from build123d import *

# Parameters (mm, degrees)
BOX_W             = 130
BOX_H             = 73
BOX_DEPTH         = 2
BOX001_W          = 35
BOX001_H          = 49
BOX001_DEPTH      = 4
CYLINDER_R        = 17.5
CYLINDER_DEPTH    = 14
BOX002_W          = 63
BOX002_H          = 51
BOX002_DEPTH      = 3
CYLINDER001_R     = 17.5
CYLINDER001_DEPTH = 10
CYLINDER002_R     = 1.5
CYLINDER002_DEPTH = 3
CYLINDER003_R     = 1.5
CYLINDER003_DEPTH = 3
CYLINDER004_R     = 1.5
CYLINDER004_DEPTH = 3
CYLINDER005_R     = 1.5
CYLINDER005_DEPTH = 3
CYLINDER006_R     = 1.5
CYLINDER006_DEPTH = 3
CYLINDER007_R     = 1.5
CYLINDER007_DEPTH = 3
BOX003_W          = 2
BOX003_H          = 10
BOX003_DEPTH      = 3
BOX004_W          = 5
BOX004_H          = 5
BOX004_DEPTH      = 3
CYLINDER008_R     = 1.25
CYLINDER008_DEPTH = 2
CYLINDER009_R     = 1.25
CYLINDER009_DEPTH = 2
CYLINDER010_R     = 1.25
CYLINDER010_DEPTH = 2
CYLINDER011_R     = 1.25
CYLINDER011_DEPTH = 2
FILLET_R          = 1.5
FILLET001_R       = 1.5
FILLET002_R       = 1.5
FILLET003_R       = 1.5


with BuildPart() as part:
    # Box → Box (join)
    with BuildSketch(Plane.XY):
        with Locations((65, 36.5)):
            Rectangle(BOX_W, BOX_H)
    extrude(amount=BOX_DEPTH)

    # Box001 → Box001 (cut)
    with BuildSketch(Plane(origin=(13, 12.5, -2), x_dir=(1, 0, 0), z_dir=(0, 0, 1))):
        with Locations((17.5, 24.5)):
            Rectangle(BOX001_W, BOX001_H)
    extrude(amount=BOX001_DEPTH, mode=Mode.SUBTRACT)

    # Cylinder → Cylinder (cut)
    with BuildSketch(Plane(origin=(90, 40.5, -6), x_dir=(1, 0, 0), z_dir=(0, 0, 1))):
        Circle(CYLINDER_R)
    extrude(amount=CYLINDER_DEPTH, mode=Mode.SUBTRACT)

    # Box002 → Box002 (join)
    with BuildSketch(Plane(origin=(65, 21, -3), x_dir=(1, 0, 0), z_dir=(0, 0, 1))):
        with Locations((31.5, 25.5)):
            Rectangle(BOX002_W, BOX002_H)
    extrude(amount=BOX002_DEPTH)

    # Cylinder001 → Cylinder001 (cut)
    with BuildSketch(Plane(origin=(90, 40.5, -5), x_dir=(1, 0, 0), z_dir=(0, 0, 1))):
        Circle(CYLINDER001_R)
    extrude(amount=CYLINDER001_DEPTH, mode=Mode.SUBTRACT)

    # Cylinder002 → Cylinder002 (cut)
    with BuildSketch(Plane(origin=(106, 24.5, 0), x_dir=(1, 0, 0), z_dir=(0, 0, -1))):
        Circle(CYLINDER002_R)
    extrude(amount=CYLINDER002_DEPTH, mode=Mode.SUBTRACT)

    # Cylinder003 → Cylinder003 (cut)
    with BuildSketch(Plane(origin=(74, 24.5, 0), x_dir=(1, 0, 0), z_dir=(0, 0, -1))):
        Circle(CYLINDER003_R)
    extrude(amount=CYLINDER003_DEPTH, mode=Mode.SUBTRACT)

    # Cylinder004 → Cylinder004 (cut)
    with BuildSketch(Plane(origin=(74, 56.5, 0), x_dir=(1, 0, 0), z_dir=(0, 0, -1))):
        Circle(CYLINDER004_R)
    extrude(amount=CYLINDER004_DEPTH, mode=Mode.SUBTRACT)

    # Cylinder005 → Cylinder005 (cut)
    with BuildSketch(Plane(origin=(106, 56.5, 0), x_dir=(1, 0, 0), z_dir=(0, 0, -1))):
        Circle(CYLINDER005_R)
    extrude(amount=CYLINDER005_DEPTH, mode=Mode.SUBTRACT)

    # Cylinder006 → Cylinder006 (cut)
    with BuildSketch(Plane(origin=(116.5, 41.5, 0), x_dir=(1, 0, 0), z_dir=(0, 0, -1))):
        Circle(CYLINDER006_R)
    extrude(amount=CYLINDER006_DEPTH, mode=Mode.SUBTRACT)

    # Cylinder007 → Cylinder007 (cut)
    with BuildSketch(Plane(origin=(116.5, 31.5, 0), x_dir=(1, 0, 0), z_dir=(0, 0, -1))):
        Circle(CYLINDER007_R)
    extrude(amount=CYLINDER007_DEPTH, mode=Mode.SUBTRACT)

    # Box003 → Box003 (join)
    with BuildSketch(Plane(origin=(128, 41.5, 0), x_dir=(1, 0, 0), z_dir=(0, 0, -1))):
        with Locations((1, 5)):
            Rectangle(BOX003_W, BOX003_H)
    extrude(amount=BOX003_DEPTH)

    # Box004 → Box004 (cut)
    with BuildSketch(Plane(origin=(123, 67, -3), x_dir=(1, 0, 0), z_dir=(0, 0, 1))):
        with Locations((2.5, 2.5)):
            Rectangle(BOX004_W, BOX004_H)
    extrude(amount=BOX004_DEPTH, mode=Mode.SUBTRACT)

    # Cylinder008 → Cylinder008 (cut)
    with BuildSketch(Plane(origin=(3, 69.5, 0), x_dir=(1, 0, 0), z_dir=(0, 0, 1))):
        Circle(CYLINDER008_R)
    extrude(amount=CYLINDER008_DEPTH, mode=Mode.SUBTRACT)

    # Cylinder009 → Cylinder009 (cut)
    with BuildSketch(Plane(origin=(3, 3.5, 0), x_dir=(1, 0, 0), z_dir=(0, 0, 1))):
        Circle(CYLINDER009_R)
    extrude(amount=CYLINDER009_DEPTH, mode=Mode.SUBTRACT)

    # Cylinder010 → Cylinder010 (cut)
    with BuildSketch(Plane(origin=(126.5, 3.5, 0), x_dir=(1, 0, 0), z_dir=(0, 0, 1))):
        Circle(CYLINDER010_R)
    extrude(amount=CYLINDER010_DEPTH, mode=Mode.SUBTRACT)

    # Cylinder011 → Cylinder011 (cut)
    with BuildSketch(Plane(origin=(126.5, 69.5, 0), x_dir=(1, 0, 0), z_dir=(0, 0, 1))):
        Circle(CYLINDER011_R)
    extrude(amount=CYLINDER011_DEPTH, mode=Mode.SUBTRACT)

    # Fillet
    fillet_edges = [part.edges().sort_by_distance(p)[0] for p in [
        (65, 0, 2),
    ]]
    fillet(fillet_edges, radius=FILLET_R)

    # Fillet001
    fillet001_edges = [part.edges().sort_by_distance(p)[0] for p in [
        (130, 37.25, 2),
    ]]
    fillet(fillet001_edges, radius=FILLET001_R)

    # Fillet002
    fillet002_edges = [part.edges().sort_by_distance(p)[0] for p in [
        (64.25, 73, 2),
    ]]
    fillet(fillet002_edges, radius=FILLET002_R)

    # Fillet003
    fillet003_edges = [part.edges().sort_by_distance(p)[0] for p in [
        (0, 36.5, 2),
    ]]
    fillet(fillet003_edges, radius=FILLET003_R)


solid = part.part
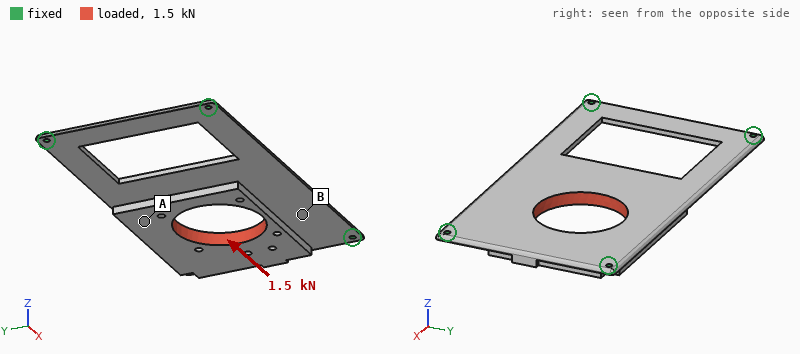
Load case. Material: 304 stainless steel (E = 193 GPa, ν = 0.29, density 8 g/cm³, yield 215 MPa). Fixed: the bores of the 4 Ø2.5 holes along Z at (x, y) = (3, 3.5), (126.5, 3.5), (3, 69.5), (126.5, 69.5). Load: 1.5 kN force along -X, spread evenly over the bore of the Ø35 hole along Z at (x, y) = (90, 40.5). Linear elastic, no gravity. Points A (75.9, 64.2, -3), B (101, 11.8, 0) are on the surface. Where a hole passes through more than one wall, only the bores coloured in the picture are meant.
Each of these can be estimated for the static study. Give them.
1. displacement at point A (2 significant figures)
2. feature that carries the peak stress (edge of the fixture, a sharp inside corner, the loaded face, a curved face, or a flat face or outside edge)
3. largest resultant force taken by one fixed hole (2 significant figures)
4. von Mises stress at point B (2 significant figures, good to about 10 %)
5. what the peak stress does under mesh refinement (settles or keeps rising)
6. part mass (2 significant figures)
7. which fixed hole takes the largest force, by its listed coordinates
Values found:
45 µm
edge of the fixture
680 N
9.4 MPa
keeps rising
160 g
(126.5, 69.5)
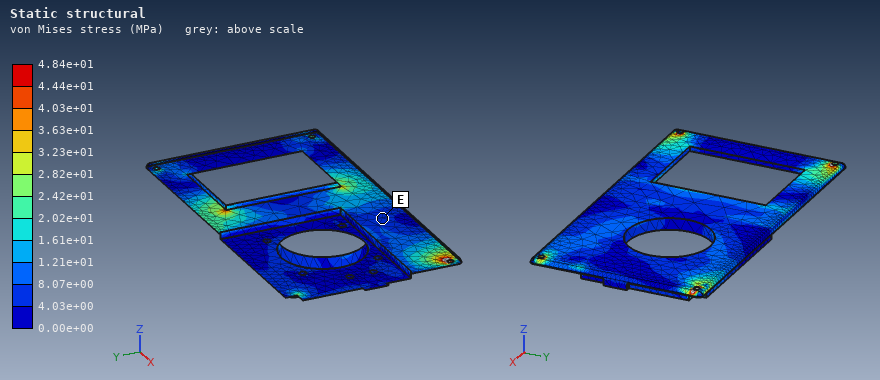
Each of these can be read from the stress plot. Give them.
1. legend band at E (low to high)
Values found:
4.03e+00 to 8.07e+00 MPa
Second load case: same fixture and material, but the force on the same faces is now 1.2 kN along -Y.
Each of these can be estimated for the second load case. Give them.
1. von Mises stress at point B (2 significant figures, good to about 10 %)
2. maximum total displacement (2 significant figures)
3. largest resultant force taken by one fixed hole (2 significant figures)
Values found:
16 MPa
12 µm
770 N
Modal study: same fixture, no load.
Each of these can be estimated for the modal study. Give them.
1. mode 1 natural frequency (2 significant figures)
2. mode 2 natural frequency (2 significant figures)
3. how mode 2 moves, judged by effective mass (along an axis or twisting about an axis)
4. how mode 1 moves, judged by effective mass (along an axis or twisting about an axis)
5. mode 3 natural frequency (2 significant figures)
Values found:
520 Hz
1200 Hz
twisting about X
along Z
2100 Hz
